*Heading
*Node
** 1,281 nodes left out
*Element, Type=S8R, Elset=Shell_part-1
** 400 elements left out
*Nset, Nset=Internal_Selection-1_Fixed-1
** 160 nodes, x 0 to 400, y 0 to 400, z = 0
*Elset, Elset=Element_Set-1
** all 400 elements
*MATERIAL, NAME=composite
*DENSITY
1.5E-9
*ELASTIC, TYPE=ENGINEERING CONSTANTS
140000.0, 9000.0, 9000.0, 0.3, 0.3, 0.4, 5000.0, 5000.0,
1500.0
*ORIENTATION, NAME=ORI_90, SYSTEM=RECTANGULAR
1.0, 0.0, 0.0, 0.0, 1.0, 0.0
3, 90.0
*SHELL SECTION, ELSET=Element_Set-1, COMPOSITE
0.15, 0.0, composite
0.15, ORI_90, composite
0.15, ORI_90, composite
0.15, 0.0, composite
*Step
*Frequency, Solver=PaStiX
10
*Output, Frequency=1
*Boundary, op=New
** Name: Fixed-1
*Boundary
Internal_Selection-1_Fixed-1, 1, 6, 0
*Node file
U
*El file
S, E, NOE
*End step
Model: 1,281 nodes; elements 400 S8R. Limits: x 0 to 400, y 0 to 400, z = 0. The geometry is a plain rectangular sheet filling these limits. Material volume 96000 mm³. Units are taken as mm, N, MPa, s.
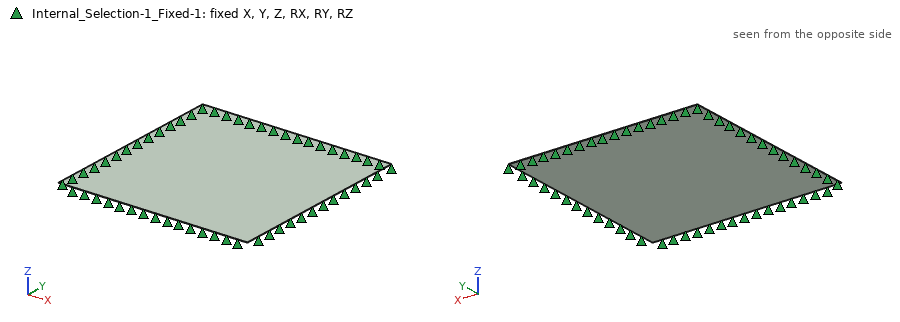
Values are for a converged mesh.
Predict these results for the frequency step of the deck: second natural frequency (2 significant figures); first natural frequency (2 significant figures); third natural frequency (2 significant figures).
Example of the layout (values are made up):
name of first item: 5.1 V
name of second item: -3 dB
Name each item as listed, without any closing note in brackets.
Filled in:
second natural frequency: 49 Hz
first natural frequency: 40 Hz
third natural frequency: 68 Hz
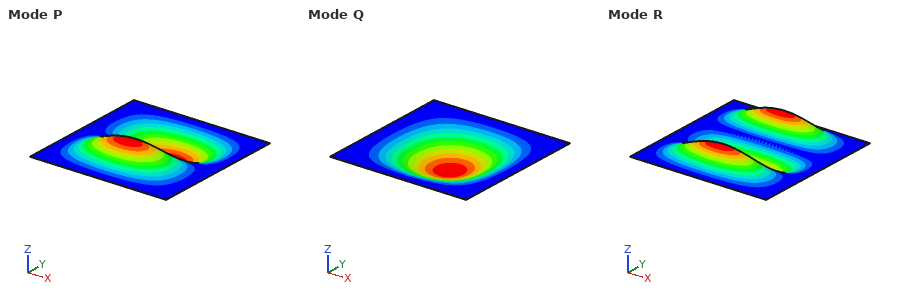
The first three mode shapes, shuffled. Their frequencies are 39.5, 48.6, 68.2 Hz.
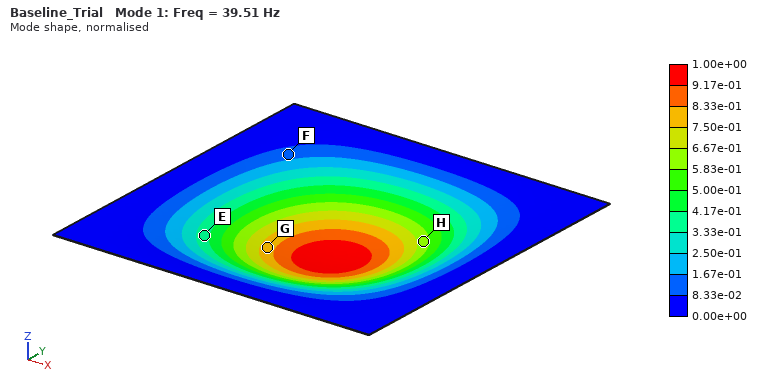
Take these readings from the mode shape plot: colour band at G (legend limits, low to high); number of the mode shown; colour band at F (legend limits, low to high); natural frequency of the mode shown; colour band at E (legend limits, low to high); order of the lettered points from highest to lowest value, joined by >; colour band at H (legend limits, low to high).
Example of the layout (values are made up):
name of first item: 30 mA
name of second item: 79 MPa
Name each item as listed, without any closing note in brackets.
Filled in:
colour band at G: 7.50e-01 to 8.33e-01
number of the mode shown: 1
colour band at F: 8.33e-02 to 1.67e-01
natural frequency of the mode shown: 39.51 Hz
colour band at E: 3.33e-01 to 4.17e-01
order of the lettered points from highest to lowest value, joined by >: G > H > E > F
colour band at H: 5.83e-01 to 6.67e-01
